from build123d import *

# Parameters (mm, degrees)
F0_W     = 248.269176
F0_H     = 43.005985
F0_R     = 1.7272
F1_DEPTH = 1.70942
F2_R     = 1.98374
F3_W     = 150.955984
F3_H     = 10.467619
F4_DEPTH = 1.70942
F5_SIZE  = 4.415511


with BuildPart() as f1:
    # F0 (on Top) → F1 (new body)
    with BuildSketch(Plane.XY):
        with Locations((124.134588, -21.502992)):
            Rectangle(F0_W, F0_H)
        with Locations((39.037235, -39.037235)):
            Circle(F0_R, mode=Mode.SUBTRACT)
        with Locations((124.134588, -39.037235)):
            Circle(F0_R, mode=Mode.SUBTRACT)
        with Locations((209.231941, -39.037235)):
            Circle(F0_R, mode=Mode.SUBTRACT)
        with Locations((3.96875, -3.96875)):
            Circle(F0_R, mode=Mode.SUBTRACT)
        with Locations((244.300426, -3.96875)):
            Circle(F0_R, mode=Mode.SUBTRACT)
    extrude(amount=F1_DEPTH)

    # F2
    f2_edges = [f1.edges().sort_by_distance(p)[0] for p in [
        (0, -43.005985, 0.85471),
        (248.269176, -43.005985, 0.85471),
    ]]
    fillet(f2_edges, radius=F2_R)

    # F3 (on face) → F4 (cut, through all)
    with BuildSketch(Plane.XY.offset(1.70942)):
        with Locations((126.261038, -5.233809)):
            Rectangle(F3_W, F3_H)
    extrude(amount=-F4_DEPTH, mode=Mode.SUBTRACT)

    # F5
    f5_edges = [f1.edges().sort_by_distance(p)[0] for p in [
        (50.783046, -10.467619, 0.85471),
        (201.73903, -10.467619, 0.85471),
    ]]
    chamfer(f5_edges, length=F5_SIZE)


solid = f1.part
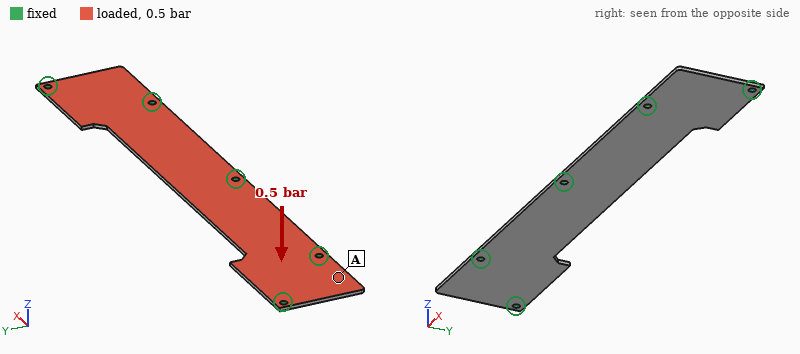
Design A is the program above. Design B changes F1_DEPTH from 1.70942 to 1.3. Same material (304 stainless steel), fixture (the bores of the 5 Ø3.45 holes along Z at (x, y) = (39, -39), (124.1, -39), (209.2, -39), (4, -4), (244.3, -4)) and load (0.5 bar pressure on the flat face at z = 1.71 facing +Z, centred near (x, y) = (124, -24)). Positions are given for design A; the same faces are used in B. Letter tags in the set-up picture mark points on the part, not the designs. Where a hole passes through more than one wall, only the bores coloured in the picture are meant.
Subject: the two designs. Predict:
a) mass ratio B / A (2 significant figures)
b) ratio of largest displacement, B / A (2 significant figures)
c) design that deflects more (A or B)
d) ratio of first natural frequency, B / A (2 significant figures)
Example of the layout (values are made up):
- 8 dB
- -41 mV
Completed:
- 0.76
- 2.2
- B
- 0.77
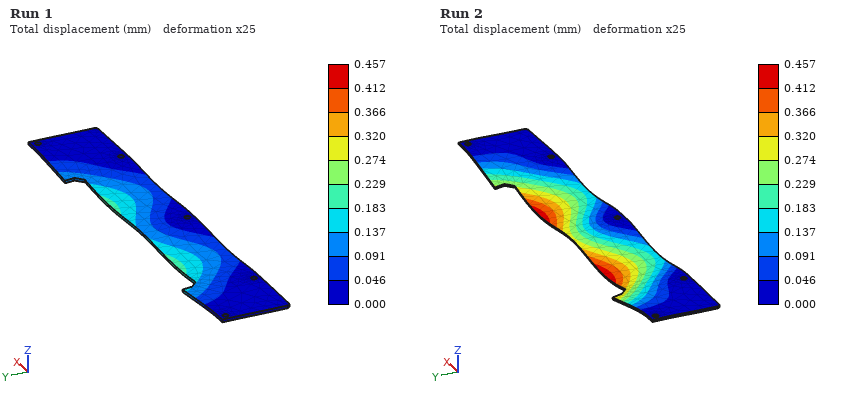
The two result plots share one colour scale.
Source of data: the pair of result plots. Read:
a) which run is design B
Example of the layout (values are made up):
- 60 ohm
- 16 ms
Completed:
- Run 2
